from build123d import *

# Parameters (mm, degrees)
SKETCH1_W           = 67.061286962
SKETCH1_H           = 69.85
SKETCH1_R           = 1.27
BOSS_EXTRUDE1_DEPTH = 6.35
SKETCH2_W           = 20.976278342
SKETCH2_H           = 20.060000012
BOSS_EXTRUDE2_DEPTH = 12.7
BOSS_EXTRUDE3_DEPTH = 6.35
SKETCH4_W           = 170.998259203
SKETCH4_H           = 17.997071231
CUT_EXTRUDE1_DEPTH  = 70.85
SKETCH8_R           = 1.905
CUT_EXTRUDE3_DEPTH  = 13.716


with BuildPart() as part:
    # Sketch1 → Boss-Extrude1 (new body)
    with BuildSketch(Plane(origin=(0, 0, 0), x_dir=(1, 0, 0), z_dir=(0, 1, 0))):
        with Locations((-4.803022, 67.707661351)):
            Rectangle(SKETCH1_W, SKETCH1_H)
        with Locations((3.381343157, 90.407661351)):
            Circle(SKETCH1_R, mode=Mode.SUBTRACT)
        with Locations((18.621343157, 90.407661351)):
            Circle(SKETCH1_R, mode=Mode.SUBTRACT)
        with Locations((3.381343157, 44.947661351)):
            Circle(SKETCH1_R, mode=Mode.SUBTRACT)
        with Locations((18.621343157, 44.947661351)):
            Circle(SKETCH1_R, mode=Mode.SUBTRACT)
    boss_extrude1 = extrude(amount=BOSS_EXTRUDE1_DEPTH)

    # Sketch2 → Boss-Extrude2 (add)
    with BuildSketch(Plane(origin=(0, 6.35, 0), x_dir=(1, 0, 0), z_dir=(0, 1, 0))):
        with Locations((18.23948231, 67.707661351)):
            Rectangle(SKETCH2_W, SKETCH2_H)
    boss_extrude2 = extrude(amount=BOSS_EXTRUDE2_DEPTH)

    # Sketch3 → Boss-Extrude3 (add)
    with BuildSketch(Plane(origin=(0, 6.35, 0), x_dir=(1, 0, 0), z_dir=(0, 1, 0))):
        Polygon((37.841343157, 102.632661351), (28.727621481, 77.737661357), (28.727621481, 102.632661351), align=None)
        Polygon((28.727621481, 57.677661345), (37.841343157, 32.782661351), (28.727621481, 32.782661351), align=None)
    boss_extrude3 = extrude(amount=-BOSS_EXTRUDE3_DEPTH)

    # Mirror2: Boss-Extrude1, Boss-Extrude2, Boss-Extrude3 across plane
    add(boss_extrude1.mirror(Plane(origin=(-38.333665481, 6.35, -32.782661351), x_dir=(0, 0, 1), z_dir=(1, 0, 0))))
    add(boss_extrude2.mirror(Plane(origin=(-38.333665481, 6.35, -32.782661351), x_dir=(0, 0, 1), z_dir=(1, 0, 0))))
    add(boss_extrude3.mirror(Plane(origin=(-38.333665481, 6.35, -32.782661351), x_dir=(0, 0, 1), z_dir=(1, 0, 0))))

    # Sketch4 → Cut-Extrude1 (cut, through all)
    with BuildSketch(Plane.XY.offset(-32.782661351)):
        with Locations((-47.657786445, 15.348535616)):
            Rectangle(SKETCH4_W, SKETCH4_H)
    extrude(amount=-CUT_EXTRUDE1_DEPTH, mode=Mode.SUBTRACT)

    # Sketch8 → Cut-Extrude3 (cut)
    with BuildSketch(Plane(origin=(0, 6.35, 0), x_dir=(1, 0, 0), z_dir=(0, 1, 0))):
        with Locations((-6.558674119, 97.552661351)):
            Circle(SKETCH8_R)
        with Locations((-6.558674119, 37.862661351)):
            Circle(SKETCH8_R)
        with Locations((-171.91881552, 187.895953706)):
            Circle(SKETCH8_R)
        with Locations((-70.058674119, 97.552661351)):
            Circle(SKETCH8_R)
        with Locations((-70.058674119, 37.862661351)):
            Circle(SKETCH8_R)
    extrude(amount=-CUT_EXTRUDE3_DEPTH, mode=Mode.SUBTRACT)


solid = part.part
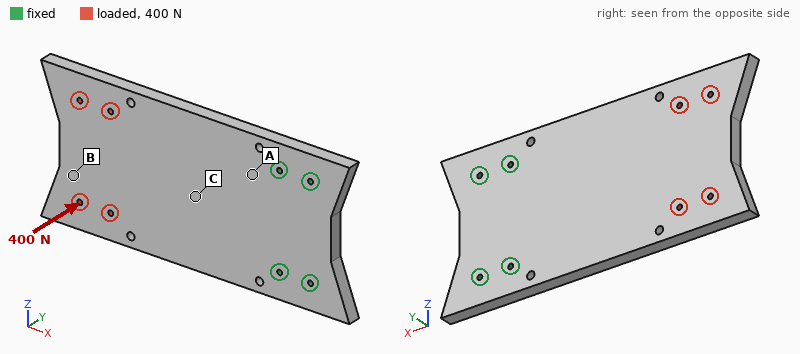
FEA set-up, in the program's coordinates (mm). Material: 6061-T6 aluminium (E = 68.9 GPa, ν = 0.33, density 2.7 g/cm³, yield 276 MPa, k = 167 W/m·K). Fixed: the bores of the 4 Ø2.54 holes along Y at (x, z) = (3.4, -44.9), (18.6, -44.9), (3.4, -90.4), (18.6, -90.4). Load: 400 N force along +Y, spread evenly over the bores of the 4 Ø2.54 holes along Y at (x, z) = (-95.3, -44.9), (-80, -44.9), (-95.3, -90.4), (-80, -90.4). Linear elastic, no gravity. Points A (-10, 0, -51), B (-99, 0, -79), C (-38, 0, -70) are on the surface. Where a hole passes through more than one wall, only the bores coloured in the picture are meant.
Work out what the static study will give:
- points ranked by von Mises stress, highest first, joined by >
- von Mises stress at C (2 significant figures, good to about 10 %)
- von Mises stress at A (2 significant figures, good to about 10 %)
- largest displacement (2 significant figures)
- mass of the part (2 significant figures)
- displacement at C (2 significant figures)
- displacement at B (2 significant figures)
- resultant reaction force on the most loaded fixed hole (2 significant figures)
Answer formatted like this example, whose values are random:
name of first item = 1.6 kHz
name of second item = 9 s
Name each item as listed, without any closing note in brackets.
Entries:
points ranked by von Mises stress, highest first, joined by > = A > C > B
von Mises stress at C = 40 MPa
von Mises stress at A = 63 MPa
largest displacement = 1.6 mm
mass of the part = 170 g
displacement at C = 0.33 mm
displacement at B = 1.3 mm
resultant reaction force on the most loaded fixed hole = 850 N
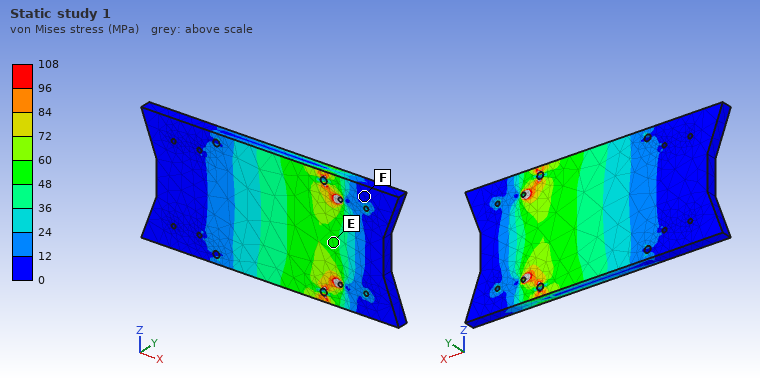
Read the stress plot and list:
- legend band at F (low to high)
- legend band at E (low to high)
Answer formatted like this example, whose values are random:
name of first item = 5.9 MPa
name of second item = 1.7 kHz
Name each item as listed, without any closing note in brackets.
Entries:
legend band at F = 0 to 12 MPa
legend band at E = 48 to 60 MPa
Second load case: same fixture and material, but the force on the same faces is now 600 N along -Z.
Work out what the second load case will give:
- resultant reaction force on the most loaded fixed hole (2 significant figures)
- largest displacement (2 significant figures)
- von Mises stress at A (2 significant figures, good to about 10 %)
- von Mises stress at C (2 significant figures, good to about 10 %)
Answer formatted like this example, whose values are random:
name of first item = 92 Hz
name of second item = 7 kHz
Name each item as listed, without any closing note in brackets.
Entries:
resultant reaction force on the most loaded fixed hole = 880 N
largest displacement = 30 µm
von Mises stress at A = 6.3 MPa
von Mises stress at C = 3.7 MPa
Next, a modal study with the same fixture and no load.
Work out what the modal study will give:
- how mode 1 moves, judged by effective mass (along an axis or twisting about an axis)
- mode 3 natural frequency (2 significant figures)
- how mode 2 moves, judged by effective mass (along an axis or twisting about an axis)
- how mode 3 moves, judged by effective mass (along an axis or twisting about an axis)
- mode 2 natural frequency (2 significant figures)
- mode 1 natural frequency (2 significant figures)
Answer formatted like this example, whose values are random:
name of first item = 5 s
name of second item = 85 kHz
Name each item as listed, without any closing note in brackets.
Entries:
how mode 1 moves, judged by effective mass = along Y
mode 3 natural frequency = 2400 Hz
how mode 2 moves, judged by effective mass = twisting about X
how mode 3 moves, judged by effective mass = along Y
mode 2 natural frequency = 1400 Hz
mode 1 natural frequency = 390 Hz
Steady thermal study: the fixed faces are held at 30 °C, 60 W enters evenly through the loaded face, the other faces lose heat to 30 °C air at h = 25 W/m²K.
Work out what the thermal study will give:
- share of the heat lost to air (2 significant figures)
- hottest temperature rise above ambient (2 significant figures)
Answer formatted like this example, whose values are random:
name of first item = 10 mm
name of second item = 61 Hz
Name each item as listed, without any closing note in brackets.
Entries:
share of the heat lost to air = 29 %
hottest temperature rise above ambient = 67 K
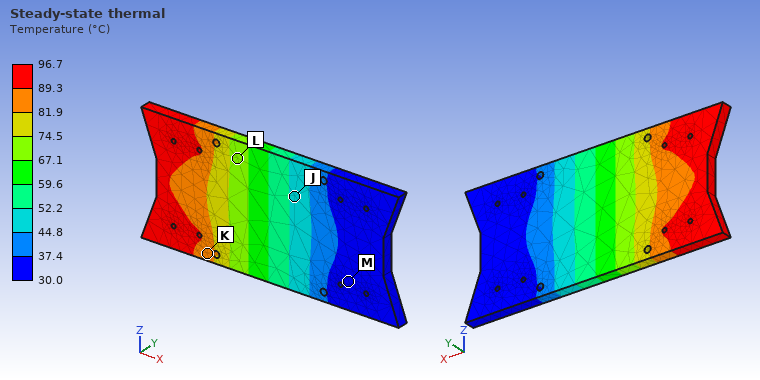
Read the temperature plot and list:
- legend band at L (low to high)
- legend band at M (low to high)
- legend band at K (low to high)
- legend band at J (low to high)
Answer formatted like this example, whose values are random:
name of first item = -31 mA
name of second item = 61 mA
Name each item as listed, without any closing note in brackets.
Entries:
legend band at L = 67.1 to 74.5 °C
legend band at M = 30.0 to 37.4 °C
legend band at K = 81.9 to 89.3 °C
legend band at J = 44.8 to 52.2 °C
